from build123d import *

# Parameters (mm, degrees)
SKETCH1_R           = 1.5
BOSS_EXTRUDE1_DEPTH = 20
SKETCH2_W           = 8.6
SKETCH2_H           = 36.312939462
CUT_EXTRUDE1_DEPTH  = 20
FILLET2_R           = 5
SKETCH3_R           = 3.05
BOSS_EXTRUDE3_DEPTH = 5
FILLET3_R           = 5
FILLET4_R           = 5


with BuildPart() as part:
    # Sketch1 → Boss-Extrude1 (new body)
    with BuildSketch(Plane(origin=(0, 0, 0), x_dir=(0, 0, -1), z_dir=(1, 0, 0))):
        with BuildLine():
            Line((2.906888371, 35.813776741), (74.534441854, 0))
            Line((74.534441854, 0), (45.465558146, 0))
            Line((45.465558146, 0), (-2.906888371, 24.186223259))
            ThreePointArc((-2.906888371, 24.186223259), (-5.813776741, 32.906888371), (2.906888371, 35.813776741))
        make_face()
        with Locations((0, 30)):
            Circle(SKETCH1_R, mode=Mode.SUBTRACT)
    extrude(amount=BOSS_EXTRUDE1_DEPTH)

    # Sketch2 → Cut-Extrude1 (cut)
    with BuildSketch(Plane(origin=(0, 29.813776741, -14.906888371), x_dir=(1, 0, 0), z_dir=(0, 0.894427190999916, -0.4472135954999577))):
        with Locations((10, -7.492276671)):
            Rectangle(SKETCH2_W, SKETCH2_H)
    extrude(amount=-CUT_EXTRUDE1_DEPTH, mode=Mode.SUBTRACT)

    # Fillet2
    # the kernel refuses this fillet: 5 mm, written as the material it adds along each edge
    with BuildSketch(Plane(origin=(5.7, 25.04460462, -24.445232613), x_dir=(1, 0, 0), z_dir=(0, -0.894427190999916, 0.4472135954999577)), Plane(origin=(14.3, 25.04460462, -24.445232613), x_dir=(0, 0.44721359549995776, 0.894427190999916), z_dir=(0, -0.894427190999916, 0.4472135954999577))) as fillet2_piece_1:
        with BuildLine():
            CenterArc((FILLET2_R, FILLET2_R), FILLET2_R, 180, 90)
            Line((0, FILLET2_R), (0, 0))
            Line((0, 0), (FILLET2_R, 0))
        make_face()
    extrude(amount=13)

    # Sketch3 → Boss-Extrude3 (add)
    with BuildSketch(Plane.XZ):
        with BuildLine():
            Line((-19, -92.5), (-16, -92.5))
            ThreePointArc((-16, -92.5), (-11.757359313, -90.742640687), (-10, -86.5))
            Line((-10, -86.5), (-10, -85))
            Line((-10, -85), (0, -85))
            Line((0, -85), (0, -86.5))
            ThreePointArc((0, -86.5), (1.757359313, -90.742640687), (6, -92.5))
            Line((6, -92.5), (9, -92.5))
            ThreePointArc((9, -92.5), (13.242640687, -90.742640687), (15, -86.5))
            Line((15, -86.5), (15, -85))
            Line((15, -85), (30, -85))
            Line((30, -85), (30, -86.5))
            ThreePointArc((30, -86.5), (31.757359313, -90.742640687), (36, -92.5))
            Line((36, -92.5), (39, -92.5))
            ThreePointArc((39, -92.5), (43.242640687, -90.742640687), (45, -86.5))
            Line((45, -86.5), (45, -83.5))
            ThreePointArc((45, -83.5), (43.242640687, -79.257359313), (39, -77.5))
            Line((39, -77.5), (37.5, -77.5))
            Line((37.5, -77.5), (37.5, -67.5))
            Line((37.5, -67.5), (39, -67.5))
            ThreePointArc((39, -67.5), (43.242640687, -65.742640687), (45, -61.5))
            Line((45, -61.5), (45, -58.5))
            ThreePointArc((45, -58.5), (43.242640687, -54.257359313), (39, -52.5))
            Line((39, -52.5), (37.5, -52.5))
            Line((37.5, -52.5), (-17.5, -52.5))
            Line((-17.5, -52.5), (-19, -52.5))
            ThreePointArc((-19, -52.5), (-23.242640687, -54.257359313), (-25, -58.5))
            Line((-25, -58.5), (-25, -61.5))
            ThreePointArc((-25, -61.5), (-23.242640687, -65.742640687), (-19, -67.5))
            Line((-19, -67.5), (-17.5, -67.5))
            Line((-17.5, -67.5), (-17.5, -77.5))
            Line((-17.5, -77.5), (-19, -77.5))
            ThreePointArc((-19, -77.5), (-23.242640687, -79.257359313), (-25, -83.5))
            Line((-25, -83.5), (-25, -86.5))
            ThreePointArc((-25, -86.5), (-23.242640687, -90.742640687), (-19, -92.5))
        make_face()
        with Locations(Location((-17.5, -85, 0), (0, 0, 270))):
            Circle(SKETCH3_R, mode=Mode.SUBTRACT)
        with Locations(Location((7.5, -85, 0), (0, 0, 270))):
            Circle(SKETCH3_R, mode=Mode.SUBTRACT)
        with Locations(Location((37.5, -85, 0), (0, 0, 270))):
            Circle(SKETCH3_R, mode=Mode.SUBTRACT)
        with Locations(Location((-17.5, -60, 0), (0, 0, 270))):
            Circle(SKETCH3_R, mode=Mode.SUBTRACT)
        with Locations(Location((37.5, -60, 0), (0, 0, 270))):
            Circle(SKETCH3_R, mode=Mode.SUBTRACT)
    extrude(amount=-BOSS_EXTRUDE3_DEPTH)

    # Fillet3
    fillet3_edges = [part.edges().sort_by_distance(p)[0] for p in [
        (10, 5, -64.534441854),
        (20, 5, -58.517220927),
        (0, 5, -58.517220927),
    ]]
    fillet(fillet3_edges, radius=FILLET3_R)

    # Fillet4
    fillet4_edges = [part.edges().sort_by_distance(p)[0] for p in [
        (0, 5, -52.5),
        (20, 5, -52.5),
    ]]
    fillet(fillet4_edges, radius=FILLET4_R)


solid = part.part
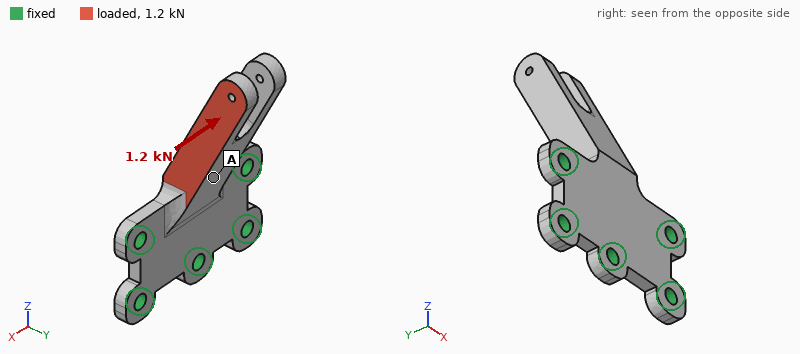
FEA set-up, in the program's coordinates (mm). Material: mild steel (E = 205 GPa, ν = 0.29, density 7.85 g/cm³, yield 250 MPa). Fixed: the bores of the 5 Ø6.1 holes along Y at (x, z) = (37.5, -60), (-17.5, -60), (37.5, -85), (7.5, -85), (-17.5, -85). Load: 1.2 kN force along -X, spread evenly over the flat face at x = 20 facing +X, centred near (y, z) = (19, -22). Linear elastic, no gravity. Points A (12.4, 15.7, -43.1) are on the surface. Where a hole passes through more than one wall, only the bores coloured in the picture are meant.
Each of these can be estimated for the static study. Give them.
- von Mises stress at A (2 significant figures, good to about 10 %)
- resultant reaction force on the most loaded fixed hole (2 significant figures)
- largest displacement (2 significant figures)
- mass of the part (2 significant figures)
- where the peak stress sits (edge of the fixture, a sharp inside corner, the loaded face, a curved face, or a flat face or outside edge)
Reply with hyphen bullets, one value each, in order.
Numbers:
- 15 MPa
- 940 N
- 0.10 mm
- 200 g
- a curved face
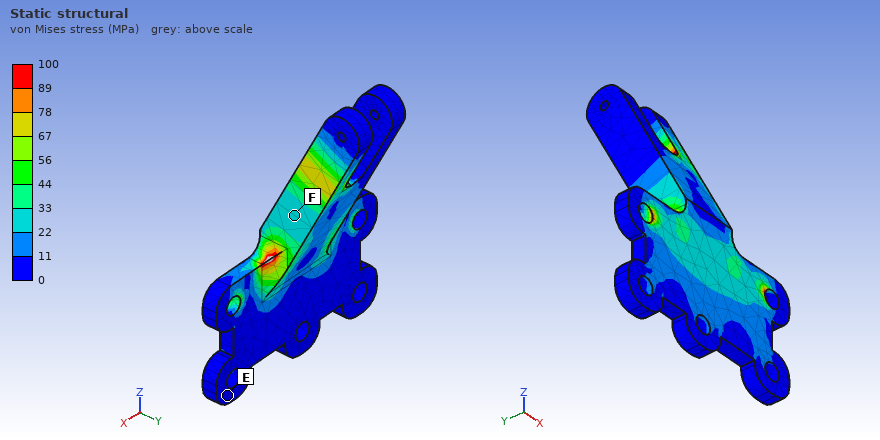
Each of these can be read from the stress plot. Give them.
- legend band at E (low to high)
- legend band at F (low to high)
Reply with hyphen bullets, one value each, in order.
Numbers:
- 0 to 11 MPa
- 22 to 33 MPa
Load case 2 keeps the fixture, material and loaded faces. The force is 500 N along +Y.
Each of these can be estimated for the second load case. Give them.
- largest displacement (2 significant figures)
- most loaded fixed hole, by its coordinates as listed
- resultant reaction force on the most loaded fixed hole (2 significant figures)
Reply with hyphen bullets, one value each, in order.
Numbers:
- 0.17 mm
- (37.5, -60)
- 760 N
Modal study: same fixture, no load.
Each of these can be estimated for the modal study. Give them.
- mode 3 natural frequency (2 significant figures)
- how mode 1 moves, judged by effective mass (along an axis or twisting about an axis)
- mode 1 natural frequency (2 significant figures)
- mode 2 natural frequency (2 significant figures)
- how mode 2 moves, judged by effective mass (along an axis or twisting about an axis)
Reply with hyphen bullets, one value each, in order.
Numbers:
- 5200 Hz
- along Y
- 1200 Hz
- 3000 Hz
- along X
